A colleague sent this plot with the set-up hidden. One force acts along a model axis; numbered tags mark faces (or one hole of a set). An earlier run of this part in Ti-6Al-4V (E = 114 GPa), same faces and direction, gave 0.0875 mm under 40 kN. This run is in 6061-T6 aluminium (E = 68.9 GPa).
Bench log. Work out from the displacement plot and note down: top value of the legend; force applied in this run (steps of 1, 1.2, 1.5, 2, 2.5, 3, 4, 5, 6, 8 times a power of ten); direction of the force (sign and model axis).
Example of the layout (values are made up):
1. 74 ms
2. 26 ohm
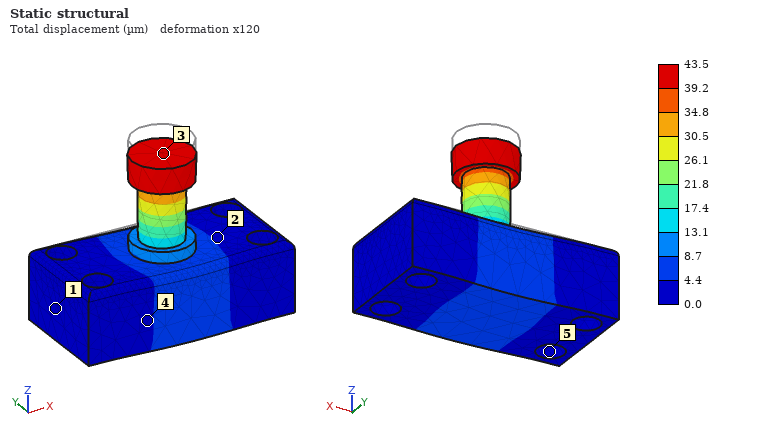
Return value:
1. 43.5 µm
2. 12 kN
3. -Z
